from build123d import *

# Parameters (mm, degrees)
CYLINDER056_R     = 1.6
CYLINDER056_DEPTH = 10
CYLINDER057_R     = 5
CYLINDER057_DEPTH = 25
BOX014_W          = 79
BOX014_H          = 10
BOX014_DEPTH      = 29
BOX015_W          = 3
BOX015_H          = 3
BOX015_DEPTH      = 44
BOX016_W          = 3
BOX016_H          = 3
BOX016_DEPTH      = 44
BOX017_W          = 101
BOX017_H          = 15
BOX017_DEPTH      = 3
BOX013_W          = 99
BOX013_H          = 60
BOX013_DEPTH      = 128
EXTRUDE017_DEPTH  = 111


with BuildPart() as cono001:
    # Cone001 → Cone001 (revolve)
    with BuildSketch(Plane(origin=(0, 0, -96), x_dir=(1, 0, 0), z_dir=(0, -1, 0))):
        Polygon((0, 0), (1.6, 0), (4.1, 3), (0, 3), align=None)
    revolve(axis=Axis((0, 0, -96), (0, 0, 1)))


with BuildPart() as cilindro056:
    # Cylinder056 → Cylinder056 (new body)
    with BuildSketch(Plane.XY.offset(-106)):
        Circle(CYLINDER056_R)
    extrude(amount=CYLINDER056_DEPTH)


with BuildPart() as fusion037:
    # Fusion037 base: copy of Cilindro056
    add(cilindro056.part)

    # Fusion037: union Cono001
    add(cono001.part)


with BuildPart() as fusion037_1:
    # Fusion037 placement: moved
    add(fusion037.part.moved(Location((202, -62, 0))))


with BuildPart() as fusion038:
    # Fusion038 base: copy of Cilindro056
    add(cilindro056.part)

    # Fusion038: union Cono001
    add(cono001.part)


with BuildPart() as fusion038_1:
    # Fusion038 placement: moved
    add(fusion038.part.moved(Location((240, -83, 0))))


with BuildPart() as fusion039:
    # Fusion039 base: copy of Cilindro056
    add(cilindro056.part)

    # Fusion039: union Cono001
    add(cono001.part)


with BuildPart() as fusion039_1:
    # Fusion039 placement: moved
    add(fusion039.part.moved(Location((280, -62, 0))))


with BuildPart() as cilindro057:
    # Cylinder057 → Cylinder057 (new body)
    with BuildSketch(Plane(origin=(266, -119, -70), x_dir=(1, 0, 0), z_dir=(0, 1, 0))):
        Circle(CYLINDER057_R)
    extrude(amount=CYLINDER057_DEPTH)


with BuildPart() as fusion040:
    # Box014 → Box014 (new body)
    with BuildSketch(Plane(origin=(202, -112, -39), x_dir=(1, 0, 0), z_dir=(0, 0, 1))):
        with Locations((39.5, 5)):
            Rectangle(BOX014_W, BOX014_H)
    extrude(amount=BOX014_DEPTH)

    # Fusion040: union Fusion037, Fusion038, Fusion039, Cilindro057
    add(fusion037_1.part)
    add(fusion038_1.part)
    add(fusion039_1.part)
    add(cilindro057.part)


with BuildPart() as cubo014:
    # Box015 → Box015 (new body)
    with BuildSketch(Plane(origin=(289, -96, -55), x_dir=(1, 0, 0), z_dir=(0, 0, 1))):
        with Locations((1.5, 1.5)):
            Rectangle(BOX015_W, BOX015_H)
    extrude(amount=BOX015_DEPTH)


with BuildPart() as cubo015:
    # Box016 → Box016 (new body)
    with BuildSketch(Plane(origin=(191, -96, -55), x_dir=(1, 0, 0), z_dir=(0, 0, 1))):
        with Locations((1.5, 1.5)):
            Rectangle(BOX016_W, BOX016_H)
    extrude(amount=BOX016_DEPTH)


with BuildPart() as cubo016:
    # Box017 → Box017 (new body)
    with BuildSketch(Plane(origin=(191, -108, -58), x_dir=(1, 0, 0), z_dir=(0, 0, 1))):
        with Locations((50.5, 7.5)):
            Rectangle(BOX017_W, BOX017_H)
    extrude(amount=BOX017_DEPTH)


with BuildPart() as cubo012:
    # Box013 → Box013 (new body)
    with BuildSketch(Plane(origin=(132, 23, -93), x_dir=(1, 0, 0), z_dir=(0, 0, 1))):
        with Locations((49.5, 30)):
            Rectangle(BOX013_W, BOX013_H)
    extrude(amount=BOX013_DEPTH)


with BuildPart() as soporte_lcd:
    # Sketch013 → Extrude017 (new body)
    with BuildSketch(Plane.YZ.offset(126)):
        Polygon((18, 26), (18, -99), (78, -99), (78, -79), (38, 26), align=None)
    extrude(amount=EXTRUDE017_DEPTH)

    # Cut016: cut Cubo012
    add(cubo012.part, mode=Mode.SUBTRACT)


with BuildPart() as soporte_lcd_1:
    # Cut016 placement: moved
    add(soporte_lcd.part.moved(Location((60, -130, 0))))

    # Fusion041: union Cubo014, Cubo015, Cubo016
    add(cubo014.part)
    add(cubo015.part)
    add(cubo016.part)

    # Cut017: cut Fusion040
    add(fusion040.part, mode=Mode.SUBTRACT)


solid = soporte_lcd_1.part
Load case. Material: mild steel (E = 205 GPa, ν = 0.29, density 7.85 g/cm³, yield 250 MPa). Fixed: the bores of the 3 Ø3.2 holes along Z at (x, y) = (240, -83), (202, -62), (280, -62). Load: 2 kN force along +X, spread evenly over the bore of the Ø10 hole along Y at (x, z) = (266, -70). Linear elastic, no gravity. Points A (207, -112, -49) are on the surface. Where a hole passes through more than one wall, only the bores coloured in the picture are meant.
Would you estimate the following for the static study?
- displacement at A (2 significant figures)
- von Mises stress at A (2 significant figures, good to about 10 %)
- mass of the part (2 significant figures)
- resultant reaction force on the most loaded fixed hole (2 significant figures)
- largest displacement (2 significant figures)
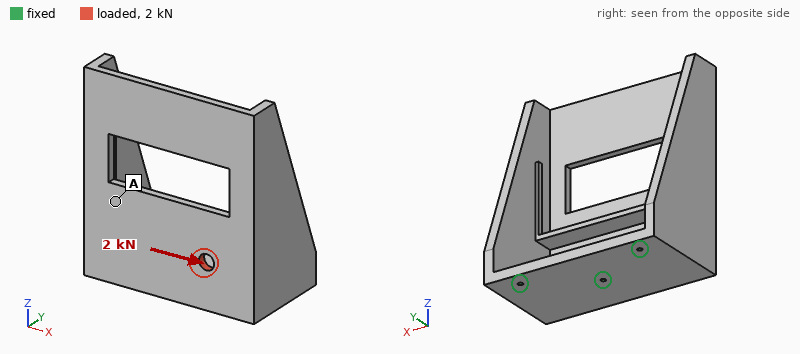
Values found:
0.059 mm
8.7 MPa
1.2 kg
1.2 kN
0.17 mm
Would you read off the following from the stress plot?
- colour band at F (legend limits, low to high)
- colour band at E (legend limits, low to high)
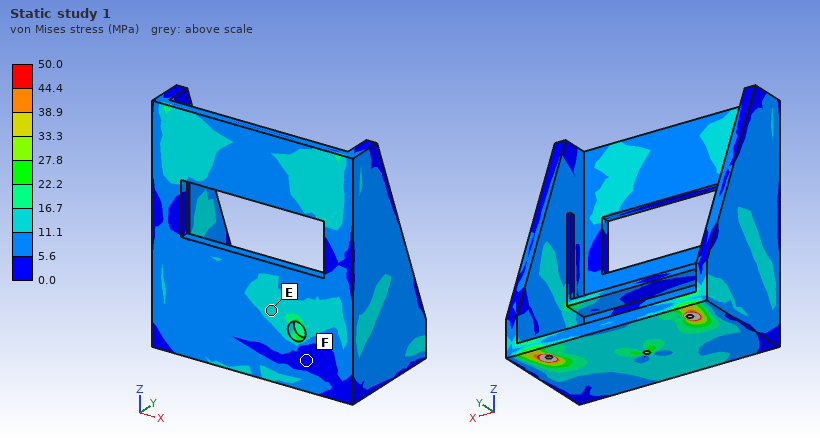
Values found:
0.0 to 5.6 MPa
11.1 to 16.7 MPa
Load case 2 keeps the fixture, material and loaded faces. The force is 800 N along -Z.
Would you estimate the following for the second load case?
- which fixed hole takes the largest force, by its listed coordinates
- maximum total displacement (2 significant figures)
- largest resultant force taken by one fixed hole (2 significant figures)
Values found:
(240, -83)
0.16 mm
1.3 kN
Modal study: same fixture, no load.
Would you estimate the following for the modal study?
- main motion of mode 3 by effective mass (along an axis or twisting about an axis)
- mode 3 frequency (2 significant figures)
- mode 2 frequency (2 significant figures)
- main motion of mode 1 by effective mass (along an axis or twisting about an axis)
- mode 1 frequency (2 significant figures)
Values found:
along Z
1600 Hz
450 Hz
along X
430 Hz
